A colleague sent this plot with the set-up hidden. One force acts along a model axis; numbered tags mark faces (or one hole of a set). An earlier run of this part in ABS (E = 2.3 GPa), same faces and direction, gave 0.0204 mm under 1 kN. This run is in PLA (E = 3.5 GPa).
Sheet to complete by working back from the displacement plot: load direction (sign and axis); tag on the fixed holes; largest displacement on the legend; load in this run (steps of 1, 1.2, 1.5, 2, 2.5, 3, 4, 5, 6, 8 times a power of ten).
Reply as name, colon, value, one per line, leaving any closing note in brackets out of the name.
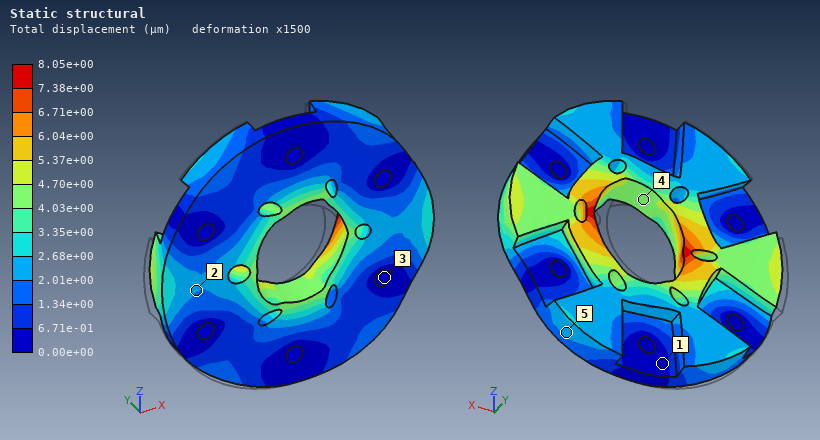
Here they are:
load direction: +X
tag on the fixed holes: 3
largest displacement on the legend: 8.05e+00 µm
load in this run: 600 N
